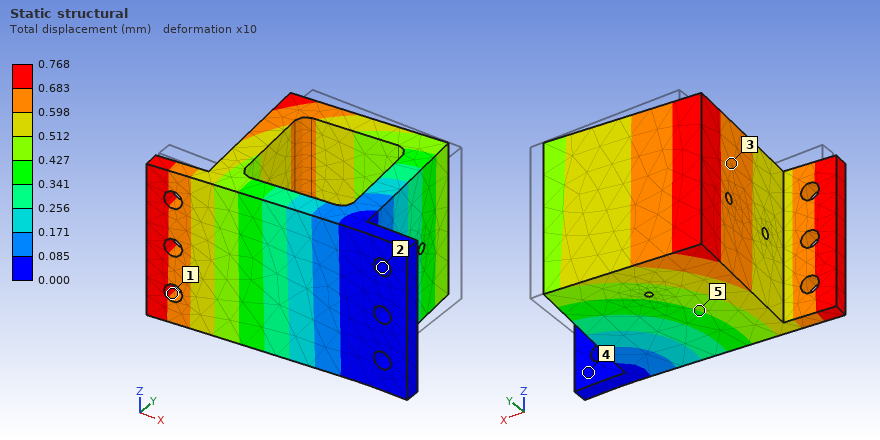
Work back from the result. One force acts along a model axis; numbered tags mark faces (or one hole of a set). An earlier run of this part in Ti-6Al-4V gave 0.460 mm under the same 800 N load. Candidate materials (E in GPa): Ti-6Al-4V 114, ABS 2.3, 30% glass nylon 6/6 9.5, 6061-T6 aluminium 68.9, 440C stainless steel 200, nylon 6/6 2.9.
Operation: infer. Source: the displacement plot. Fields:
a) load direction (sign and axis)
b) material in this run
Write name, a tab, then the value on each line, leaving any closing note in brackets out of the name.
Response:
load direction	-Y
material in this run	6061-T6 aluminium
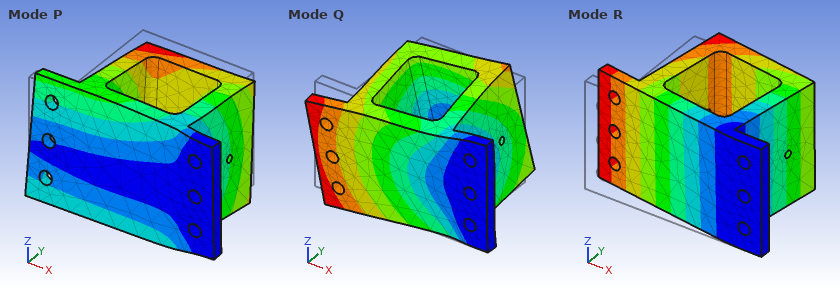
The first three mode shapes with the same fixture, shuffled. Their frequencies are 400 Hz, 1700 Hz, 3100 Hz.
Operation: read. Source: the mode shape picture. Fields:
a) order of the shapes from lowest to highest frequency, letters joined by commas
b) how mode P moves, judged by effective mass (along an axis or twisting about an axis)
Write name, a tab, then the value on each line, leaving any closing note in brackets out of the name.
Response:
order of the shapes from lowest to highest frequency, letters joined by commas	R, P, Q
how mode P moves, judged by effective mass	along Z
